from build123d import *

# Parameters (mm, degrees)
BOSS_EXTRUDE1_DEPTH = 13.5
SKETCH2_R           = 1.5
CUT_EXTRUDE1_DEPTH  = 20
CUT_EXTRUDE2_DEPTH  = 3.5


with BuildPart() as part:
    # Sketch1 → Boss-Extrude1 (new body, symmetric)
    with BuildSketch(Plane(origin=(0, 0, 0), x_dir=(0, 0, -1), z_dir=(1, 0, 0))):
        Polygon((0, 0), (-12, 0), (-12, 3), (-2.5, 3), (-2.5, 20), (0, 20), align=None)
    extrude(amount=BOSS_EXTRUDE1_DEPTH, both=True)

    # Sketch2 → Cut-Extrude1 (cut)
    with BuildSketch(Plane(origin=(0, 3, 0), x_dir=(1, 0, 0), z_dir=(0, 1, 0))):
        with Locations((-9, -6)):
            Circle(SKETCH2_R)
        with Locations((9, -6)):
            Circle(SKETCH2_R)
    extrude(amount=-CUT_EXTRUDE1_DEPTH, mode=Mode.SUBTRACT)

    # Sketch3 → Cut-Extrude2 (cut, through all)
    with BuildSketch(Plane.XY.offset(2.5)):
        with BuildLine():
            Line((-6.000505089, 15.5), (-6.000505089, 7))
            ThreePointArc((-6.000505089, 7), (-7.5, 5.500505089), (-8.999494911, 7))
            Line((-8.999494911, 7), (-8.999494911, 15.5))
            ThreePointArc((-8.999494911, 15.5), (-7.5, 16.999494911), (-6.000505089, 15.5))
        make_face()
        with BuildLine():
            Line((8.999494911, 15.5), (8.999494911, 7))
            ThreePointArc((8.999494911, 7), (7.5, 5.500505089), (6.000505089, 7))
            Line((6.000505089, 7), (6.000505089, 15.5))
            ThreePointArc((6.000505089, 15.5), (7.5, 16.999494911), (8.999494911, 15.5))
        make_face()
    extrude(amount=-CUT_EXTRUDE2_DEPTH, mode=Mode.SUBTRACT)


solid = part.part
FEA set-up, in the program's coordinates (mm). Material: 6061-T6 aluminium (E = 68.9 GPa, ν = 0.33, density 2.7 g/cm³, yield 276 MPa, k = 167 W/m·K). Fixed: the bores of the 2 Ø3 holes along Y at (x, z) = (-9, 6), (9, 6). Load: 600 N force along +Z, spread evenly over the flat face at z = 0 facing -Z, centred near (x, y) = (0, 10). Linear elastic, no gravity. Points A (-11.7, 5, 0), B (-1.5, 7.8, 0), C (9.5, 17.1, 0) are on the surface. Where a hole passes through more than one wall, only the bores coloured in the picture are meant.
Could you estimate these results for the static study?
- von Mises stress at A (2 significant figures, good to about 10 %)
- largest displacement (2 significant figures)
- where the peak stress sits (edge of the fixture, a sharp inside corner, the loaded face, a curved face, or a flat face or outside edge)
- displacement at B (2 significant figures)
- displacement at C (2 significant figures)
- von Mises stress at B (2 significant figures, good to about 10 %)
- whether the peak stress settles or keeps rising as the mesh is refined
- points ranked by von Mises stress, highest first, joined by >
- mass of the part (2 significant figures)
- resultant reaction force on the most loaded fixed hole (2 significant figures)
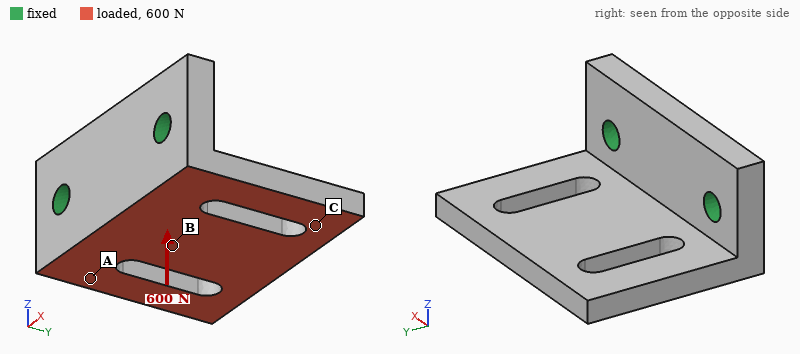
130 MPa
0.27 mm
edge of the fixture
0.069 mm
0.22 mm
86 MPa
keeps rising
A > B > C
5.2 g
300 N
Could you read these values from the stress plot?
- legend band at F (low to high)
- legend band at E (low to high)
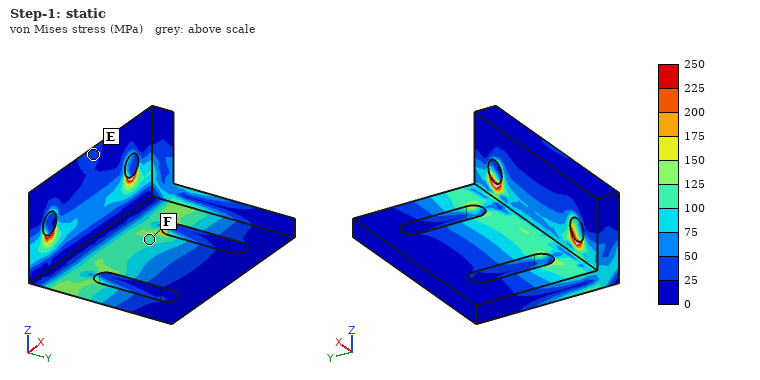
100 to 125 MPa
25 to 50 MPa
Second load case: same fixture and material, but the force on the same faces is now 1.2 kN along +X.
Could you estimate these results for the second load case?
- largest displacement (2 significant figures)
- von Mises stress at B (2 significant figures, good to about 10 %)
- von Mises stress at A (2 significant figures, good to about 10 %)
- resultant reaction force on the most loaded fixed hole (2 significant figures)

43 µm
43 MPa
24 MPa
850 N
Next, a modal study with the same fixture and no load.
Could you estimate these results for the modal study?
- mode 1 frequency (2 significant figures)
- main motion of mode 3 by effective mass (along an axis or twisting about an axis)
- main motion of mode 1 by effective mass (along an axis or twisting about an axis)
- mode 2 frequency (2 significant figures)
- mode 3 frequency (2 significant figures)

5100 Hz
along X
along Z
9500 Hz
18 kHz
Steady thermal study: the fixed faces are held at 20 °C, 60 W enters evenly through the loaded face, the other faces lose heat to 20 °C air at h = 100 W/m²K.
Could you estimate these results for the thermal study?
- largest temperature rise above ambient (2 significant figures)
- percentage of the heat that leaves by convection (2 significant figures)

68 K
7.0 %
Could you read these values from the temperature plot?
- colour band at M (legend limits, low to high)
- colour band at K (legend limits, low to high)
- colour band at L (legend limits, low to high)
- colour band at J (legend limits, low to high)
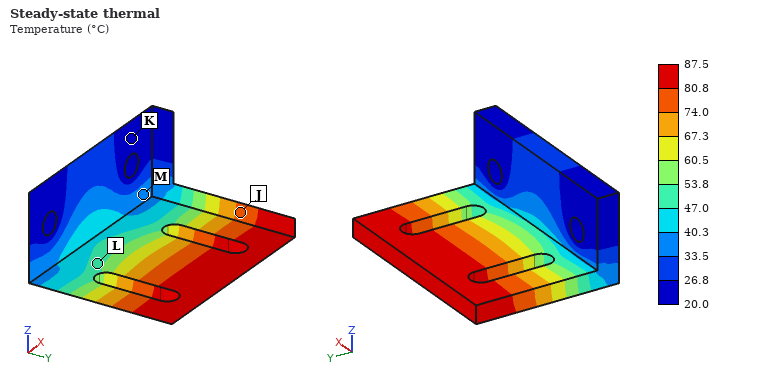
33.5 to 40.3 °C
20.0 to 26.8 °C
47.0 to 53.8 °C
74.0 to 80.8 °C
